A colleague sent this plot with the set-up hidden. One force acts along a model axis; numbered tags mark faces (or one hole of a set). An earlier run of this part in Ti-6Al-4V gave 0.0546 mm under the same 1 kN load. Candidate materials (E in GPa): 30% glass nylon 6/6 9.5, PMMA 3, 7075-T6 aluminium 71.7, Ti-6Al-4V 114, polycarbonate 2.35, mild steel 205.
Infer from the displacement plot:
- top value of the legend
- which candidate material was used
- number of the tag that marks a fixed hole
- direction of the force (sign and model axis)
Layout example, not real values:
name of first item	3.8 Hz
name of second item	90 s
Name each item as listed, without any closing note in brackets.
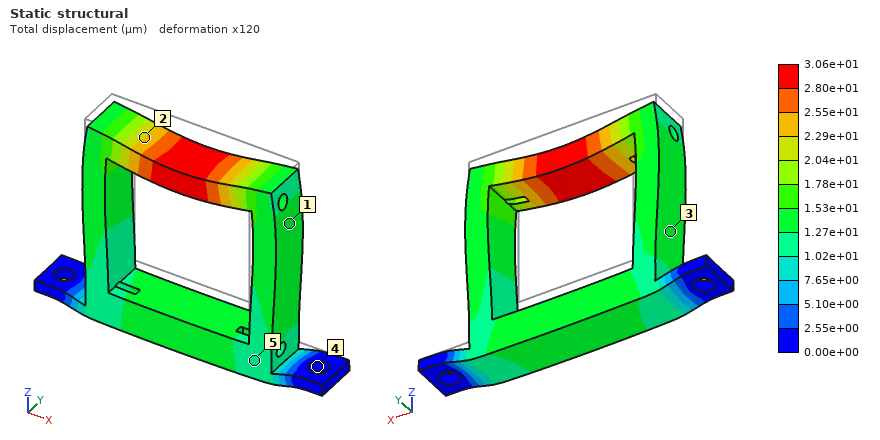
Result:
top value of the legend	3.06e+01 µm
which candidate material was used	mild steel
number of the tag that marks a fixed hole	4
direction of the force	-Z
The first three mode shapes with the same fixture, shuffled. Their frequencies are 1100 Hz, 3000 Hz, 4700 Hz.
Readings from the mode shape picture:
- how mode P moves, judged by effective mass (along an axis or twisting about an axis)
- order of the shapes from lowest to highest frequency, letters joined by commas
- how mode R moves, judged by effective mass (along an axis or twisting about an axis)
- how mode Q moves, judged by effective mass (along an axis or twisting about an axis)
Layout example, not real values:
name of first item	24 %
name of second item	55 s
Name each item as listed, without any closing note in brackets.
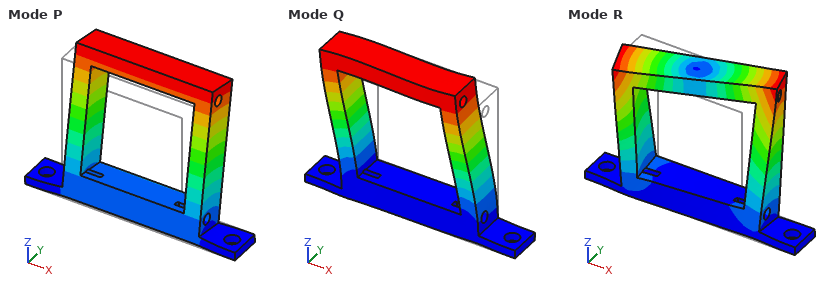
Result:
how mode P moves, judged by effective mass	along Y
order of the shapes from lowest to highest frequency, letters joined by commas	P, Q, R
how mode R moves, judged by effective mass	twisting about Z
how mode Q moves, judged by effective mass	along X
